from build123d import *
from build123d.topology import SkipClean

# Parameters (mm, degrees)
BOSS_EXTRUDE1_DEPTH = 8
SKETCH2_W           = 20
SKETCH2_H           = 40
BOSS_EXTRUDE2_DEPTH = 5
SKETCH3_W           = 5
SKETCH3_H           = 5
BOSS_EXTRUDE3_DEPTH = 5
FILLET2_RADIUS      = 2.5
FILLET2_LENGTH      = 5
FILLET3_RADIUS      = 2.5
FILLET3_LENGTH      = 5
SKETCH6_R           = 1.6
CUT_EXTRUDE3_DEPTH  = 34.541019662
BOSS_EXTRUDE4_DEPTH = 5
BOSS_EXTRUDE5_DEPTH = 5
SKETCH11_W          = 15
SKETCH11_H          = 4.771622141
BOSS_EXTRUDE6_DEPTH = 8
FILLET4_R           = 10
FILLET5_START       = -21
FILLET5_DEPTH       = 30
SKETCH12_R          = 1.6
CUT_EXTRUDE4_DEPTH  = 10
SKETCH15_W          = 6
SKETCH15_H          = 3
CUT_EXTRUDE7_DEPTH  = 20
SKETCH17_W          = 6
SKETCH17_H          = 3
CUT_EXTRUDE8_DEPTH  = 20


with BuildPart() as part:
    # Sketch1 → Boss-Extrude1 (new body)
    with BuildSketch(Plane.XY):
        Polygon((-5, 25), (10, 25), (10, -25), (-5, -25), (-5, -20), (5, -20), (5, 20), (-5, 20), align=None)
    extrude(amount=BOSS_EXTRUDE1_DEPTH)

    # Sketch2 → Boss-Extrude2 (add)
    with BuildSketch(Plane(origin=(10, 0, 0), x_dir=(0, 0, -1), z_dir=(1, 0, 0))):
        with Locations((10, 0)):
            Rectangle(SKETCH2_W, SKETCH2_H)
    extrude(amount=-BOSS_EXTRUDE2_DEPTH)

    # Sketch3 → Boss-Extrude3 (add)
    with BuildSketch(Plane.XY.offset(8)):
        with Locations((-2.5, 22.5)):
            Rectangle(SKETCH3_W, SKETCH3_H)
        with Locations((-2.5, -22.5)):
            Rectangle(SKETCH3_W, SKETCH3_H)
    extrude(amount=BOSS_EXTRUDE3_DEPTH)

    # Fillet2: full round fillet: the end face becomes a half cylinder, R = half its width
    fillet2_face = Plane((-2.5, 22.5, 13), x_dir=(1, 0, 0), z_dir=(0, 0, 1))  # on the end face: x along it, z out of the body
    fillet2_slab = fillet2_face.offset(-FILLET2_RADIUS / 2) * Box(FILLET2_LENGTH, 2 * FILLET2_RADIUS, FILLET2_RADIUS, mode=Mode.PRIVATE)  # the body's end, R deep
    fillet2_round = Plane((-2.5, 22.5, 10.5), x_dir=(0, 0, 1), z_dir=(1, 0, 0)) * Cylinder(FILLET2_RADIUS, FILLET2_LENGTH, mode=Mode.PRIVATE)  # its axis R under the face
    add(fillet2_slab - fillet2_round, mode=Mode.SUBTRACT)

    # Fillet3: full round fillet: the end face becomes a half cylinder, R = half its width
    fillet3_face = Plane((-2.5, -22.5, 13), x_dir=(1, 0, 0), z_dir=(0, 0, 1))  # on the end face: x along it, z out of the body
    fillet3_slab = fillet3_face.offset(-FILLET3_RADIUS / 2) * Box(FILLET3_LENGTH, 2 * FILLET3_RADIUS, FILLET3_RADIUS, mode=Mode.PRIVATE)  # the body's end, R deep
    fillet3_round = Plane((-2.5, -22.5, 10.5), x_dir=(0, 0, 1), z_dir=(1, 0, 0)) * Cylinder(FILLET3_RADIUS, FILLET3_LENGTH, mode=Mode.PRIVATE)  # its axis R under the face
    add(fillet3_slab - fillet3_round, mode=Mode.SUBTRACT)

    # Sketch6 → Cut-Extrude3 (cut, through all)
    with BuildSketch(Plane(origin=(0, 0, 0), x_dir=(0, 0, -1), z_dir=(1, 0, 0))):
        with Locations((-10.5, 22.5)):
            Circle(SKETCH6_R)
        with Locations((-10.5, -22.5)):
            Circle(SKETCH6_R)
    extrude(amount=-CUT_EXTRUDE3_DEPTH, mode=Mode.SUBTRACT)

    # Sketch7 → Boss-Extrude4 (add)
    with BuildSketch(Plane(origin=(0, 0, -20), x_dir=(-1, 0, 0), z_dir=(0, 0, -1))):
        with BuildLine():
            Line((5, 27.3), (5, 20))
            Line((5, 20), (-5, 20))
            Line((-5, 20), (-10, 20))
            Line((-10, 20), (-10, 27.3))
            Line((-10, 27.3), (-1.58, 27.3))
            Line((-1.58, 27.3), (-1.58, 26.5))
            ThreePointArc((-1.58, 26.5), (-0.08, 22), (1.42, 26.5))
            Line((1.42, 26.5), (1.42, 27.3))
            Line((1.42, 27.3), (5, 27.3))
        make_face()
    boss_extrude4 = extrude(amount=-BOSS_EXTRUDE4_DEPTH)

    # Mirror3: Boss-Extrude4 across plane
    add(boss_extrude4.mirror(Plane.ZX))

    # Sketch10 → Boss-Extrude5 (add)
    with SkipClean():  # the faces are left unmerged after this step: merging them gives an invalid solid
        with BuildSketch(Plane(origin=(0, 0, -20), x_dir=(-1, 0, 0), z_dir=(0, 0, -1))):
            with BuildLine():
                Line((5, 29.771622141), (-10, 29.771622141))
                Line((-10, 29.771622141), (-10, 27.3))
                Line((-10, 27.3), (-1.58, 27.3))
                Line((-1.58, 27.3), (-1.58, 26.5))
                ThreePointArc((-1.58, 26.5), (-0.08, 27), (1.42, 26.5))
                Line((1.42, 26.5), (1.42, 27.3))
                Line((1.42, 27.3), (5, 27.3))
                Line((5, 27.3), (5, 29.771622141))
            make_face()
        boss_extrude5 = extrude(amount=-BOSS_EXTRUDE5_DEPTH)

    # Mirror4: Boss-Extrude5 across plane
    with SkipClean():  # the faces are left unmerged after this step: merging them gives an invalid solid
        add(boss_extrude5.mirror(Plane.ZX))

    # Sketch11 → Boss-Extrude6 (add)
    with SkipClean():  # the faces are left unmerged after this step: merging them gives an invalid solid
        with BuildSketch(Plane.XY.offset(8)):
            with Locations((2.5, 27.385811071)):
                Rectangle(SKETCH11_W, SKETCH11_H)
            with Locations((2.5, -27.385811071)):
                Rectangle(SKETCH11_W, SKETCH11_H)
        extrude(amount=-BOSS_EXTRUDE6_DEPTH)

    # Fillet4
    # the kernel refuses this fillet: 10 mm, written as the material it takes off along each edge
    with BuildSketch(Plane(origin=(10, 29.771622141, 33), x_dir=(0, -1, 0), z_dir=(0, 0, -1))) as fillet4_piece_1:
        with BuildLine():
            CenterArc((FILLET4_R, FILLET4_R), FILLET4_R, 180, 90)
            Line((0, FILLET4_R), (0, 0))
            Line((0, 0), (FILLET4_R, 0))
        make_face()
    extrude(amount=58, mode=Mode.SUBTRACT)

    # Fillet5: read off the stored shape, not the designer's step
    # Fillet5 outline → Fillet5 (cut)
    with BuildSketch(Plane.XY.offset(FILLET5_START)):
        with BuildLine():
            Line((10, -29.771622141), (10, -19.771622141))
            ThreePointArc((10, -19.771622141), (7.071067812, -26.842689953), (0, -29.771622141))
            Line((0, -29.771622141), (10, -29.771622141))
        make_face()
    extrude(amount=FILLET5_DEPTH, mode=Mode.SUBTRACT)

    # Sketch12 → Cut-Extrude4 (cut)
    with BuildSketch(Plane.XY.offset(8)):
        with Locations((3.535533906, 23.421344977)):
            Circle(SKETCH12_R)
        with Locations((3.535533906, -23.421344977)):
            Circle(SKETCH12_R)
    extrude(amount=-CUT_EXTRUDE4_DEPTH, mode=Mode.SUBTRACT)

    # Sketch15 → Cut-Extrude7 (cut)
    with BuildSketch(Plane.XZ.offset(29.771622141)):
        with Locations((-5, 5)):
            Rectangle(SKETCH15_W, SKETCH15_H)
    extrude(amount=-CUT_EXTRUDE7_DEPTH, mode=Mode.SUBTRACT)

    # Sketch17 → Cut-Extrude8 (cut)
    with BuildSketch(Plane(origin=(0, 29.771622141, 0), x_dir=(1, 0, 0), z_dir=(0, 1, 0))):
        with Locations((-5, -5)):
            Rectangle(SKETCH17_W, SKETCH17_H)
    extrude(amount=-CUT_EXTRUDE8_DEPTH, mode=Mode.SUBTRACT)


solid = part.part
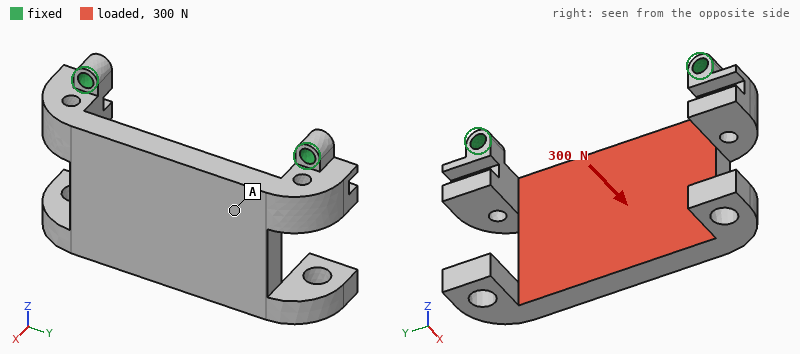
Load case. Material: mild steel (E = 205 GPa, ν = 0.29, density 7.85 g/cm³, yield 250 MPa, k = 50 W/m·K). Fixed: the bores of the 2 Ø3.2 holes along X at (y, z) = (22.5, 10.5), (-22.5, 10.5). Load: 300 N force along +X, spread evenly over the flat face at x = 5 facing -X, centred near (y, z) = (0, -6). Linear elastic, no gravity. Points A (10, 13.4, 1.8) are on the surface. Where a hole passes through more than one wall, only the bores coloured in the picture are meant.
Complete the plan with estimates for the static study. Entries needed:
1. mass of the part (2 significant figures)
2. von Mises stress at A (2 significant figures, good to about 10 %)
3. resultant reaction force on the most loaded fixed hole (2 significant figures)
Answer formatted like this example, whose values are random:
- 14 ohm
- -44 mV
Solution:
- 67 g
- 17 MPa
- 170 N
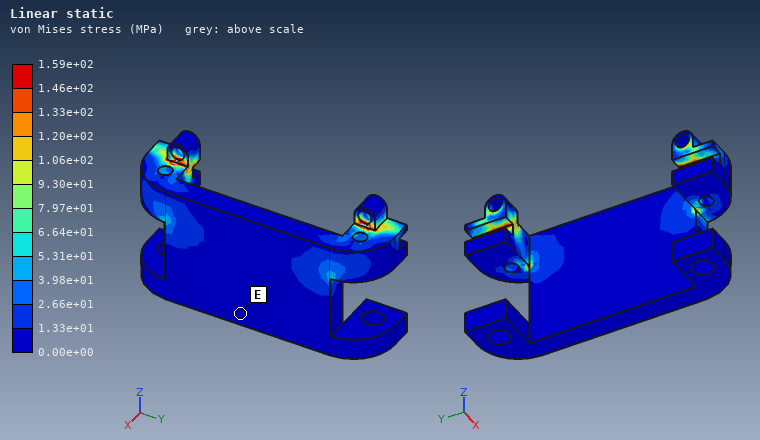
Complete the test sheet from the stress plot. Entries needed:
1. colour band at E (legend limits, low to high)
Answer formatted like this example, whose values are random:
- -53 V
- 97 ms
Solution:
- 0.00e+00 to 1.33e+01 MPa
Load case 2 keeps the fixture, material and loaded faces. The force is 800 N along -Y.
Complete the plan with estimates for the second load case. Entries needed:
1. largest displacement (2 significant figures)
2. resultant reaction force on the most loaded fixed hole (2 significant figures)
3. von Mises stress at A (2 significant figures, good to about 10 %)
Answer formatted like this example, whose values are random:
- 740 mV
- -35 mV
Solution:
- 32 µm
- 450 N
- 25 MPa
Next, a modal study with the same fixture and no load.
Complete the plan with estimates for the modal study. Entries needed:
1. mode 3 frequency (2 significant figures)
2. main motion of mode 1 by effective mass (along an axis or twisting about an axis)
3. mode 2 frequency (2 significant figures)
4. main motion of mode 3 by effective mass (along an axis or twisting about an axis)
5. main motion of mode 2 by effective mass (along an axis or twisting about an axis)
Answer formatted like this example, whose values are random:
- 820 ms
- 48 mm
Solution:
- 5800 Hz
- along X
- 3500 Hz
- along Z
- along Y
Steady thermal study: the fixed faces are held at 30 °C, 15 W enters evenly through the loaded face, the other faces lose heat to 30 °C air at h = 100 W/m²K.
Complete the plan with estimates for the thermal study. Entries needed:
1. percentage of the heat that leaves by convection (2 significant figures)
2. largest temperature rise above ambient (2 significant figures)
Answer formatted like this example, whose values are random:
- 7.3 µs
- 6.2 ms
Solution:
- 64 %
- 37 K
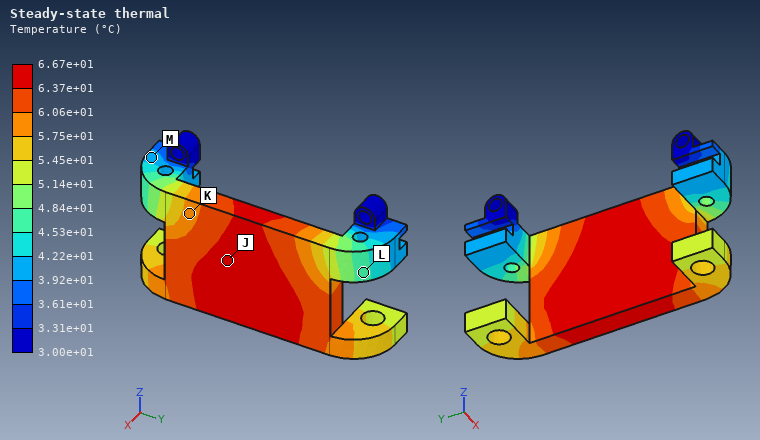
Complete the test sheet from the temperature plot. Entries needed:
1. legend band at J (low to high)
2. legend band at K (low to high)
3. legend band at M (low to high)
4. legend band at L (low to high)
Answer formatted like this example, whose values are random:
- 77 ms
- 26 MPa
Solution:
- 6.37e+01 to 6.67e+01 °C
- 5.75e+01 to 6.06e+01 °C
- 3.92e+01 to 4.22e+01 °C
- 4.53e+01 to 4.84e+01 °C
